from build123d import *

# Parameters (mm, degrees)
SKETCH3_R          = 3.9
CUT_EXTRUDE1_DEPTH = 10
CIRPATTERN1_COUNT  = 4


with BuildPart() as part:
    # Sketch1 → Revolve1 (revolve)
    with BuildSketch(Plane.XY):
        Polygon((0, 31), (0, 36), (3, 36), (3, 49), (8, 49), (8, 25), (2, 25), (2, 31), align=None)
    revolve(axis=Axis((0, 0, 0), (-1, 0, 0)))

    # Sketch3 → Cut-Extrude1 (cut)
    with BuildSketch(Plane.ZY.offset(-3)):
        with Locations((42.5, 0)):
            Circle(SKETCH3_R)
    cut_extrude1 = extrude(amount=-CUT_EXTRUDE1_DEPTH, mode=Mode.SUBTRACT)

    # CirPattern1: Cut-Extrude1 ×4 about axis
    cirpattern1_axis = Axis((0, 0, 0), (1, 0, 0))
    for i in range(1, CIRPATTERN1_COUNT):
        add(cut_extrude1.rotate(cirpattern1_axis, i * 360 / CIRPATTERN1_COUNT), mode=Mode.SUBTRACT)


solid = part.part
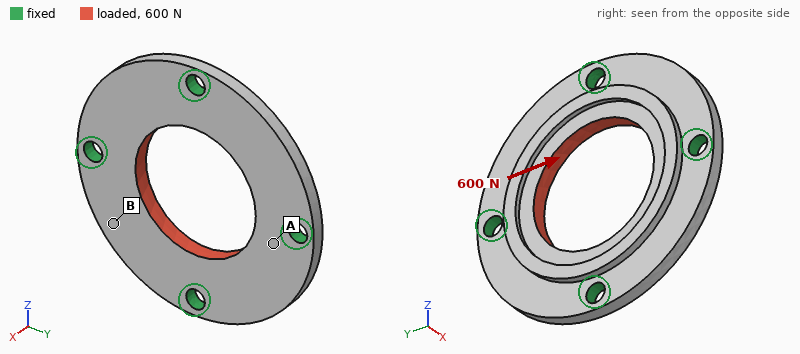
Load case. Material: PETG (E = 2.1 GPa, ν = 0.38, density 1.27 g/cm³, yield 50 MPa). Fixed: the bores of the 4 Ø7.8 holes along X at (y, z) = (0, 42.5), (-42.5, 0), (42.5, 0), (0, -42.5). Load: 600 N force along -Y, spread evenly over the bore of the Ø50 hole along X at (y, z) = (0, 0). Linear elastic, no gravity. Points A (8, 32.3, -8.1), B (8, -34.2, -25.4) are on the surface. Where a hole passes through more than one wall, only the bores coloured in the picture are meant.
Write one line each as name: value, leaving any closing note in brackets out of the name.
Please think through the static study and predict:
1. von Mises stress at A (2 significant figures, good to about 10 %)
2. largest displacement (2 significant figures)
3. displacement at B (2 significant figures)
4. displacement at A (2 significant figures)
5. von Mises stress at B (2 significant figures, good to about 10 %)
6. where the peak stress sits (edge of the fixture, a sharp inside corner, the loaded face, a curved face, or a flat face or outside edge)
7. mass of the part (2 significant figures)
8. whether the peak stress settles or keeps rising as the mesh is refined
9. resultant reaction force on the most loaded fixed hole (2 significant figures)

von Mises stress at A: 1.2 MPa
largest displacement: 21 µm
displacement at B: 16 µm
displacement at A: 8.7 µm
von Mises stress at B: 0.50 MPa
where the peak stress sits: edge of the fixture
mass of the part: 40 g
whether the peak stress settles or keeps rising as the mesh is refined: keeps rising
resultant reaction force on the most loaded fixed hole: 150 N
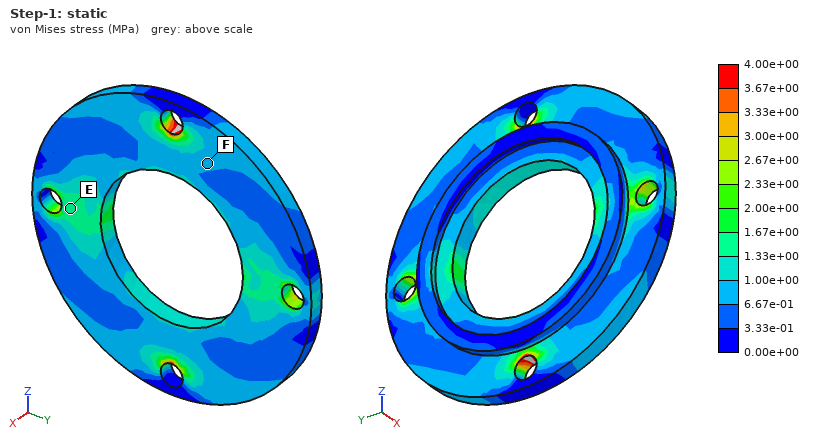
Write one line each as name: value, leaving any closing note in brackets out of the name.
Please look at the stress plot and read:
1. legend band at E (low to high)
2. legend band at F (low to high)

legend band at E: 1.33e+00 to 1.67e+00 MPa
legend band at F: 6.67e-01 to 1.00e+00 MPa
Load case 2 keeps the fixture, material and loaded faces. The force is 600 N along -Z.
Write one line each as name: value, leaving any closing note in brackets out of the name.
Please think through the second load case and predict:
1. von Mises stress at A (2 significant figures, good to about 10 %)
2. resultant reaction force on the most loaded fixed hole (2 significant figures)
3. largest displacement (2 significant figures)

von Mises stress at A: 0.77 MPa
resultant reaction force on the most loaded fixed hole: 150 N
largest displacement: 21 µm
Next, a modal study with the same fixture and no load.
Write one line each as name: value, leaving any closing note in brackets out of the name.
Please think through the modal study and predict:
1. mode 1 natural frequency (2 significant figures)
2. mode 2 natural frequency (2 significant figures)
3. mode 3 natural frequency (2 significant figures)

mode 1 natural frequency: 1700 Hz
mode 2 natural frequency: 1900 Hz
mode 3 natural frequency: 1900 Hz
